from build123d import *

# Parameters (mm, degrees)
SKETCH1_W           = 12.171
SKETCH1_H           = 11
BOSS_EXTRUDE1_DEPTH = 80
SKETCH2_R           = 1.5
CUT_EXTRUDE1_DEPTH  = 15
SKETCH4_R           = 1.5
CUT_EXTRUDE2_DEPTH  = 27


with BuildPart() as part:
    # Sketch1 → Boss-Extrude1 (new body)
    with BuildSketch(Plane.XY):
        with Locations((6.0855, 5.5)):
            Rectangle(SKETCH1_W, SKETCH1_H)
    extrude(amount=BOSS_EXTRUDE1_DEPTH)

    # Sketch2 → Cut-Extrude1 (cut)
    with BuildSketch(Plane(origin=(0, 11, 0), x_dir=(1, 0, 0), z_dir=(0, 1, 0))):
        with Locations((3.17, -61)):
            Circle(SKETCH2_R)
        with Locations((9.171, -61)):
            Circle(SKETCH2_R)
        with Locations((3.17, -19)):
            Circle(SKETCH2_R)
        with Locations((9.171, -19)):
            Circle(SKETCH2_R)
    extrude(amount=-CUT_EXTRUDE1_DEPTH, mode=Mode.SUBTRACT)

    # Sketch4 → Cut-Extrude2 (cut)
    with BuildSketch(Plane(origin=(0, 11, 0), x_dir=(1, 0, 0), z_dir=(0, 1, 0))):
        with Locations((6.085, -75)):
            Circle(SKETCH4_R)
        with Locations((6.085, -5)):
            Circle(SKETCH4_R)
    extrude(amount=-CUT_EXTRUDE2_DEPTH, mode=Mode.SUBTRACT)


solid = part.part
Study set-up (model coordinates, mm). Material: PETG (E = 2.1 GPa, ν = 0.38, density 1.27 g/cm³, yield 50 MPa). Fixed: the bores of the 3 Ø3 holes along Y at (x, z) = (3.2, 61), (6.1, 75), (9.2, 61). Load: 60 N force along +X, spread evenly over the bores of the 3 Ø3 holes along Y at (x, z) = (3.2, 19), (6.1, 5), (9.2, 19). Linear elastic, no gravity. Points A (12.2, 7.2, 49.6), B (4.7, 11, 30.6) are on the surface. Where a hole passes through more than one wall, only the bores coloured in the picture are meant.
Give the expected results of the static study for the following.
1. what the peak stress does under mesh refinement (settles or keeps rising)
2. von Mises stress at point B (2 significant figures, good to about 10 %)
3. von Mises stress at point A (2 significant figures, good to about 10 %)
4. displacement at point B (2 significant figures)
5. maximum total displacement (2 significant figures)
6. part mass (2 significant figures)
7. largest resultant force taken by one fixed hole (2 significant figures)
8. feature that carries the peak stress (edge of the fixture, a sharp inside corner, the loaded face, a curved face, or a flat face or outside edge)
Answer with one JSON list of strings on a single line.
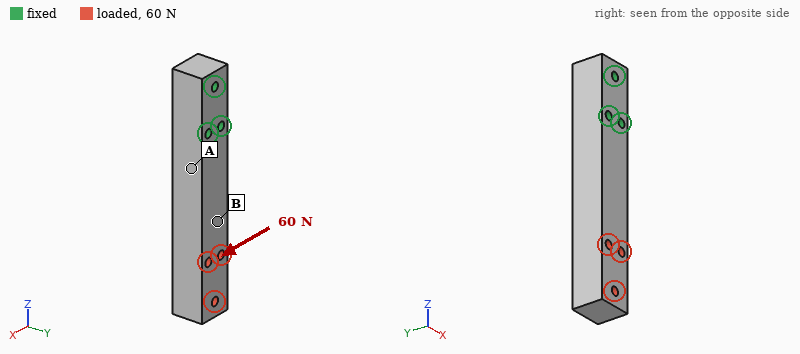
["keeps rising", "1.5 MPa", "7.8 MPa", "0.30 mm", "0.89 mm", "13 g", "340 N", "edge of the fixture"]
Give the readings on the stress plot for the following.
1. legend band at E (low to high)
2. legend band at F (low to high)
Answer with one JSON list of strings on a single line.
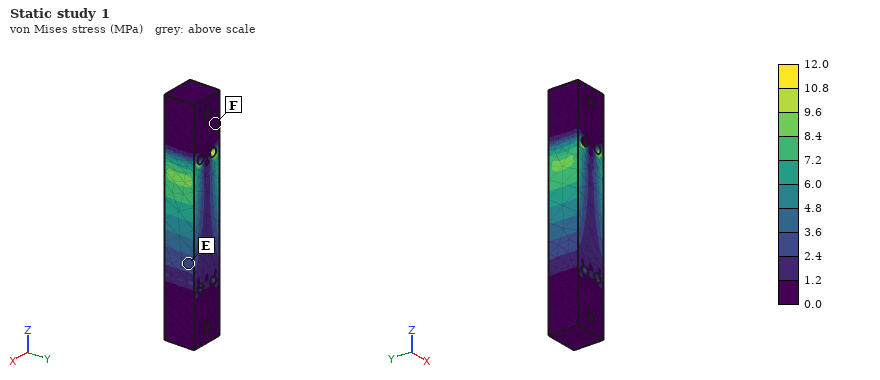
["2.4 to 3.6 MPa", "0.0 to 1.2 MPa"]
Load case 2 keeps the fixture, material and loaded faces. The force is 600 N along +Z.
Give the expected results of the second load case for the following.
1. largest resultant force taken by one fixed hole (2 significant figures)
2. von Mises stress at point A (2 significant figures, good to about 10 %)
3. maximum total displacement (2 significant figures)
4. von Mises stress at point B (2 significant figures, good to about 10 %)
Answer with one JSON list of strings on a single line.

["300 N", "4.6 MPa", "0.11 mm", "4.4 MPa"]
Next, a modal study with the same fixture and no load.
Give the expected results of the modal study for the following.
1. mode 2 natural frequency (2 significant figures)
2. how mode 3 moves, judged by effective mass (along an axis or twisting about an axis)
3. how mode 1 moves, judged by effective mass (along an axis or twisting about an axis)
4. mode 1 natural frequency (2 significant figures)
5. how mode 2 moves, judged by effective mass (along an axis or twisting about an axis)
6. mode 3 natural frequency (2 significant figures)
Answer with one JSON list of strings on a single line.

["680 Hz", "twisting about Z", "along Y", "630 Hz", "along X", "3000 Hz"]
